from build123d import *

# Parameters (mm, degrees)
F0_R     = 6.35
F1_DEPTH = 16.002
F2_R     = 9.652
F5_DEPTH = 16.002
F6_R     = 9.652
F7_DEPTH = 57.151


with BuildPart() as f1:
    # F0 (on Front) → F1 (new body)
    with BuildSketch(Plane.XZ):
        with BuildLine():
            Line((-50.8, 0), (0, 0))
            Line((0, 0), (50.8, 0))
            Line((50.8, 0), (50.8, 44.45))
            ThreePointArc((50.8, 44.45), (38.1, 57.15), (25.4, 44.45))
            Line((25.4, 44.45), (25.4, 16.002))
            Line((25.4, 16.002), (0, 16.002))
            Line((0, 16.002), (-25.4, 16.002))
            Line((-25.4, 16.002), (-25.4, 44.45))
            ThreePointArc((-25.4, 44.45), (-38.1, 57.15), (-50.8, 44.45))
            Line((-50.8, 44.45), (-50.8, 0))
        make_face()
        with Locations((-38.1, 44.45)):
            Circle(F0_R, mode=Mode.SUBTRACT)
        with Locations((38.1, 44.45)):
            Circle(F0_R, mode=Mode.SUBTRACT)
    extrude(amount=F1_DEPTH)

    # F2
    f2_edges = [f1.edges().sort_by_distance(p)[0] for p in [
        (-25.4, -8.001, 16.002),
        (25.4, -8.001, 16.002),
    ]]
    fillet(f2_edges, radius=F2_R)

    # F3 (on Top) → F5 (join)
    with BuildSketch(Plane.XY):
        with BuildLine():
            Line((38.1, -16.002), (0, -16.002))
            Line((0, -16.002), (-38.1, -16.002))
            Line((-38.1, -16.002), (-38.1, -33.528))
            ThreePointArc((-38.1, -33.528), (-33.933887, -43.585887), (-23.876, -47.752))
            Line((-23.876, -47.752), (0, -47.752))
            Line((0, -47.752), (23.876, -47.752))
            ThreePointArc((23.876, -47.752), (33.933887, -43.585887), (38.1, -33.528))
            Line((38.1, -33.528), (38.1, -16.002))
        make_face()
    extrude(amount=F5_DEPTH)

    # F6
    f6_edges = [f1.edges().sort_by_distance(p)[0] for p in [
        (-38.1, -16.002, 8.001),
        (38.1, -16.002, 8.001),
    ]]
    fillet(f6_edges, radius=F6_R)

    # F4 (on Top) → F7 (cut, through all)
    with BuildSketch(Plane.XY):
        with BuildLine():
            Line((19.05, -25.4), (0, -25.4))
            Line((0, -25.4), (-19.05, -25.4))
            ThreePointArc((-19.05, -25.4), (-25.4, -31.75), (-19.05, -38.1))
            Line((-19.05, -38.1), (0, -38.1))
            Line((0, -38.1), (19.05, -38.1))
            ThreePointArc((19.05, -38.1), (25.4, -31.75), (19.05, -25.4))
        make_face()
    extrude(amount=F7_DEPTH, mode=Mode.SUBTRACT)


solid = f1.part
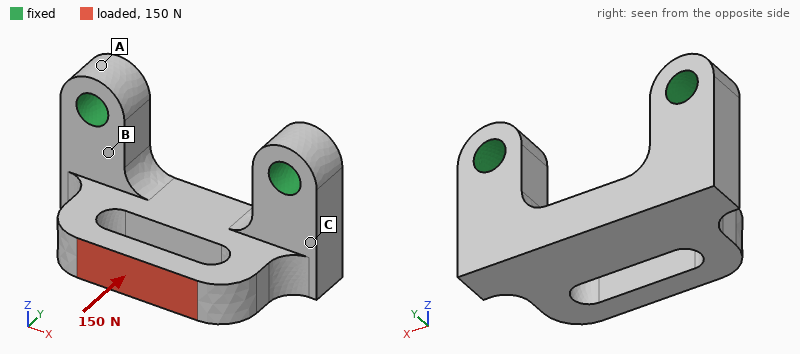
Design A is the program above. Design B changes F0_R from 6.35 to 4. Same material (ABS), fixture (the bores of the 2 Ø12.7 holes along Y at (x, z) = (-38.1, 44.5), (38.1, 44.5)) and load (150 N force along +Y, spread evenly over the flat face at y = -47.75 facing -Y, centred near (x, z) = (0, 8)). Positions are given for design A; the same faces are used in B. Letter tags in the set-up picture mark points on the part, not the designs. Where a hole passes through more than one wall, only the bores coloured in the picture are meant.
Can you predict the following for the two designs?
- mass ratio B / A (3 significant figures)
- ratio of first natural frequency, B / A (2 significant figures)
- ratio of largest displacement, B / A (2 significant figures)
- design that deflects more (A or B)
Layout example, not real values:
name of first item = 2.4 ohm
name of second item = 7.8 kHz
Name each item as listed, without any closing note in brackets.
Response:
mass ratio B / A = 1.03
ratio of first natural frequency, B / A = 0.91
ratio of largest displacement, B / A = 1.2
design that deflects more = B
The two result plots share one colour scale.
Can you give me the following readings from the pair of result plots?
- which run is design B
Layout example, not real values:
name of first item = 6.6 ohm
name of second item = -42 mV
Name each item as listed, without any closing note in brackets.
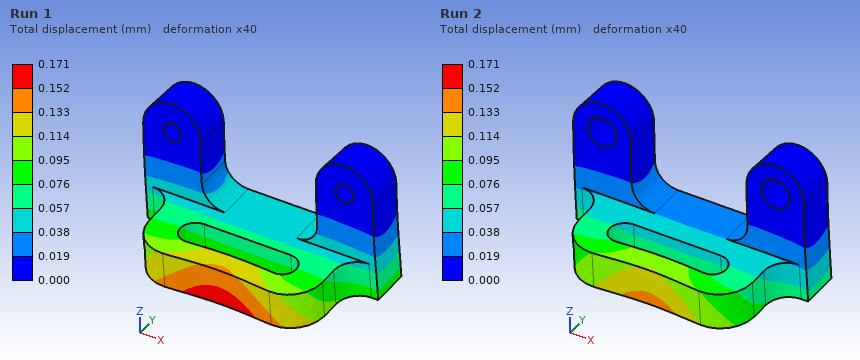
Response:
which run is design B = Run 1
